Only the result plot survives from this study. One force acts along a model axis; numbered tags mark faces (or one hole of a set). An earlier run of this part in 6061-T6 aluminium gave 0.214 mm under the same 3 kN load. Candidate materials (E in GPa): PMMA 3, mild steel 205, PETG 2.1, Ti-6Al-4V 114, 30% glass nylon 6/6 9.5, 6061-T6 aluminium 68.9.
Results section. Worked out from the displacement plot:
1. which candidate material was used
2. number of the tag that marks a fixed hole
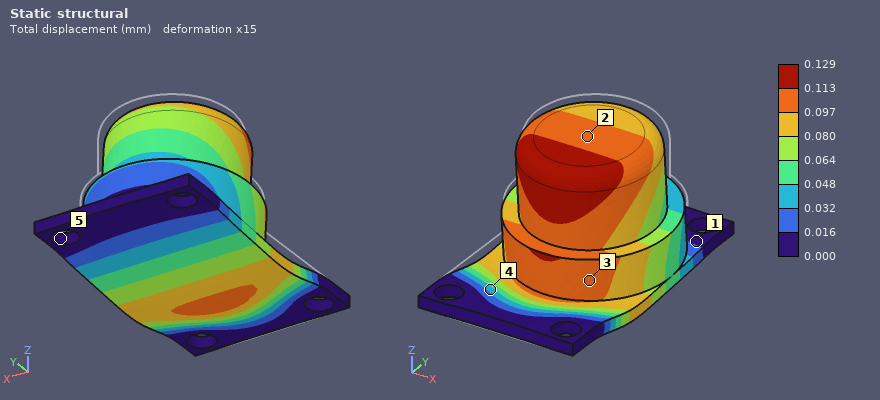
Ti-6Al-4V
5
